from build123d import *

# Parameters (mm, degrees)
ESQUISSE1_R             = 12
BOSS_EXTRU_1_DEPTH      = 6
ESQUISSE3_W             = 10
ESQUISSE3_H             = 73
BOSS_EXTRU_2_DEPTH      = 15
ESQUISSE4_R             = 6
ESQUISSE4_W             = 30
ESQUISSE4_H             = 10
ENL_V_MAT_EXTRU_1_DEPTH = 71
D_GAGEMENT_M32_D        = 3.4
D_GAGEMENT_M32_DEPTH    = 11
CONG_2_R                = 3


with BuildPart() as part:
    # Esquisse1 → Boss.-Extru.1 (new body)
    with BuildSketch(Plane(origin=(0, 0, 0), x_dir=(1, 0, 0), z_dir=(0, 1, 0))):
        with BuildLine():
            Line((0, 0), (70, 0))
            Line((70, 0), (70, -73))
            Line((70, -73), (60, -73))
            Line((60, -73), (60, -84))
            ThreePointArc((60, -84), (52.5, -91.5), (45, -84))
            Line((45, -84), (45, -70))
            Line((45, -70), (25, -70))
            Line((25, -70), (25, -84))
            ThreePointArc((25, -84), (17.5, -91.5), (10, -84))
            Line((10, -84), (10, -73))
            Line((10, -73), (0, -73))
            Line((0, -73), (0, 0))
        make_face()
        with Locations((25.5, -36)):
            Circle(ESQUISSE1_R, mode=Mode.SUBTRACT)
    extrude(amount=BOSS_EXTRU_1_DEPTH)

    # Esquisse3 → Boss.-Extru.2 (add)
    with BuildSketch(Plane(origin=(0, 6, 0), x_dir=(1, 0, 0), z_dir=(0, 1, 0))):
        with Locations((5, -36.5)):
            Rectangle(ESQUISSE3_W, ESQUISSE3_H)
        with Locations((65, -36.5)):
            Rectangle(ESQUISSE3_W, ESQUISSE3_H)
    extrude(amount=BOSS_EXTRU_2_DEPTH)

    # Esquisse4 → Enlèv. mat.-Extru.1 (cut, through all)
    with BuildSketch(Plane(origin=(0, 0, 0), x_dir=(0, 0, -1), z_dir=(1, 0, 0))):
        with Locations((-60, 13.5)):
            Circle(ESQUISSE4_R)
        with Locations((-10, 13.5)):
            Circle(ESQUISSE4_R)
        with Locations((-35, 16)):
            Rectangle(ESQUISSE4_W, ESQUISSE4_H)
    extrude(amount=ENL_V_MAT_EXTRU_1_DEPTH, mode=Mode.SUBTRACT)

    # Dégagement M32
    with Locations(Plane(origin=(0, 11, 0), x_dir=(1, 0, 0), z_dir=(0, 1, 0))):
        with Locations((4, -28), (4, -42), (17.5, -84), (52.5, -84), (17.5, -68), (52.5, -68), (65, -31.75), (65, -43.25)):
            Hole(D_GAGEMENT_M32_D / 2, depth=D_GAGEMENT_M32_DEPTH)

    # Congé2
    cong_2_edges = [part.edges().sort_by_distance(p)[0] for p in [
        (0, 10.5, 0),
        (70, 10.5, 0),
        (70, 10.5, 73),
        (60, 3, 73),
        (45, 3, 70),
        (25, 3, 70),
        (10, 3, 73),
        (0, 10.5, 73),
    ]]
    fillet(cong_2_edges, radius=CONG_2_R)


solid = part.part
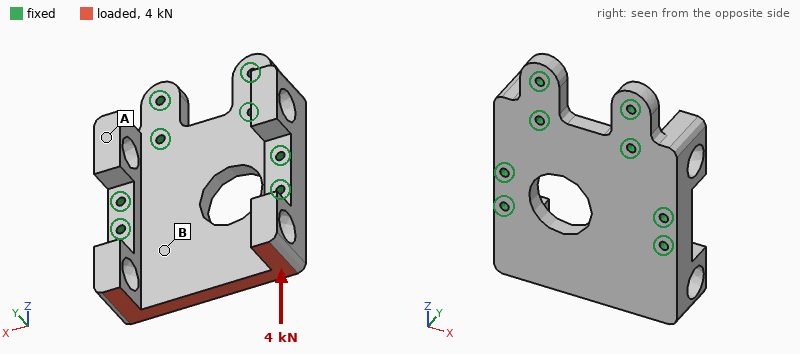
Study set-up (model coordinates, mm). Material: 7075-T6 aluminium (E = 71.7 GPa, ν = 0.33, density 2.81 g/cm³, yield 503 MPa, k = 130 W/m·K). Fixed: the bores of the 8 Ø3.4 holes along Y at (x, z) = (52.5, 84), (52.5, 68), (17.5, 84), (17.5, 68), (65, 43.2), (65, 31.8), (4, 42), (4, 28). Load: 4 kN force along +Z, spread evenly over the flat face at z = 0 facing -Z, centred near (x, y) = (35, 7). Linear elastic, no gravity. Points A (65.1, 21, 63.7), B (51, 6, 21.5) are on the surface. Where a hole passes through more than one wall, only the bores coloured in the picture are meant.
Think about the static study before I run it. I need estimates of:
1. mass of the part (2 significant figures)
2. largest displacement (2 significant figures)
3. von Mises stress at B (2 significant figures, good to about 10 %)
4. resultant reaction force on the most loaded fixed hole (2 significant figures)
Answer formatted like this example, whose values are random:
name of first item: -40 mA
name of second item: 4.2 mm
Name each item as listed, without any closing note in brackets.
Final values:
mass of the part: 120 g
largest displacement: 35 µm
von Mises stress at B: 13 MPa
resultant reaction force on the most loaded fixed hole: 1.5 kN
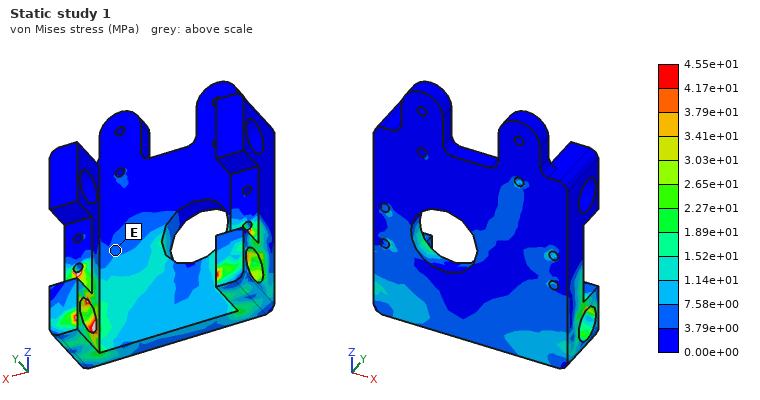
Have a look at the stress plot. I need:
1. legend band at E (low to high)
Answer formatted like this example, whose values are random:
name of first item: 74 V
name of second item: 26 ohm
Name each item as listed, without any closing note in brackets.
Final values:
legend band at E: 3.79e+00 to 7.58e+00 MPa
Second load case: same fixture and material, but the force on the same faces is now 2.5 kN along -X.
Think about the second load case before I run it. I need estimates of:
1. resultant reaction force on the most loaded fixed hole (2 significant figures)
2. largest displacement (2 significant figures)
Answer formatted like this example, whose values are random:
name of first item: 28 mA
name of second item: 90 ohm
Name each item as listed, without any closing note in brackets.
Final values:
resultant reaction force on the most loaded fixed hole: 1.6 kN
largest displacement: 44 µm
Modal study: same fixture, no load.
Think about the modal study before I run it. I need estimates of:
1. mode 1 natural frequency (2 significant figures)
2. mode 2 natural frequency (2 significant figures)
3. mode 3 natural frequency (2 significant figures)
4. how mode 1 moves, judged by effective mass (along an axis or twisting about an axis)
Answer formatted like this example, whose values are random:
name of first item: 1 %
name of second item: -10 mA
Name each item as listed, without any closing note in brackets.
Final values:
mode 1 natural frequency: 5100 Hz
mode 2 natural frequency: 7400 Hz
mode 3 natural frequency: 8900 Hz
how mode 1 moves, judged by effective mass: along Y
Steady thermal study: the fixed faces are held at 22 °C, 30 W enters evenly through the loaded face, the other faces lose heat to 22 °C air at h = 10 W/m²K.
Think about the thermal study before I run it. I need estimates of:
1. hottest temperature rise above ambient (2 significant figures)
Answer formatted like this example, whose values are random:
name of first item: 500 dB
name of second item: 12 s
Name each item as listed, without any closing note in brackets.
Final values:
hottest temperature rise above ambient: 19 K
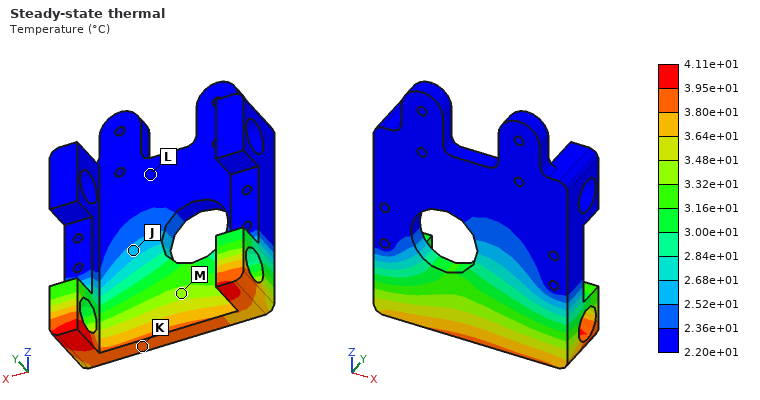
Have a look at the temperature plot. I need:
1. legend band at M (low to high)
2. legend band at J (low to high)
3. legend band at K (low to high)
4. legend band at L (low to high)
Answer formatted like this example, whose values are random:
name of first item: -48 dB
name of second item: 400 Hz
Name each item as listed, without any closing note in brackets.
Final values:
legend band at M: 3.32e+01 to 3.48e+01 °C
legend band at J: 2.52e+01 to 2.68e+01 °C
legend band at K: 3.80e+01 to 3.95e+01 °C
legend band at L: 2.20e+01 to 2.36e+01 °C
